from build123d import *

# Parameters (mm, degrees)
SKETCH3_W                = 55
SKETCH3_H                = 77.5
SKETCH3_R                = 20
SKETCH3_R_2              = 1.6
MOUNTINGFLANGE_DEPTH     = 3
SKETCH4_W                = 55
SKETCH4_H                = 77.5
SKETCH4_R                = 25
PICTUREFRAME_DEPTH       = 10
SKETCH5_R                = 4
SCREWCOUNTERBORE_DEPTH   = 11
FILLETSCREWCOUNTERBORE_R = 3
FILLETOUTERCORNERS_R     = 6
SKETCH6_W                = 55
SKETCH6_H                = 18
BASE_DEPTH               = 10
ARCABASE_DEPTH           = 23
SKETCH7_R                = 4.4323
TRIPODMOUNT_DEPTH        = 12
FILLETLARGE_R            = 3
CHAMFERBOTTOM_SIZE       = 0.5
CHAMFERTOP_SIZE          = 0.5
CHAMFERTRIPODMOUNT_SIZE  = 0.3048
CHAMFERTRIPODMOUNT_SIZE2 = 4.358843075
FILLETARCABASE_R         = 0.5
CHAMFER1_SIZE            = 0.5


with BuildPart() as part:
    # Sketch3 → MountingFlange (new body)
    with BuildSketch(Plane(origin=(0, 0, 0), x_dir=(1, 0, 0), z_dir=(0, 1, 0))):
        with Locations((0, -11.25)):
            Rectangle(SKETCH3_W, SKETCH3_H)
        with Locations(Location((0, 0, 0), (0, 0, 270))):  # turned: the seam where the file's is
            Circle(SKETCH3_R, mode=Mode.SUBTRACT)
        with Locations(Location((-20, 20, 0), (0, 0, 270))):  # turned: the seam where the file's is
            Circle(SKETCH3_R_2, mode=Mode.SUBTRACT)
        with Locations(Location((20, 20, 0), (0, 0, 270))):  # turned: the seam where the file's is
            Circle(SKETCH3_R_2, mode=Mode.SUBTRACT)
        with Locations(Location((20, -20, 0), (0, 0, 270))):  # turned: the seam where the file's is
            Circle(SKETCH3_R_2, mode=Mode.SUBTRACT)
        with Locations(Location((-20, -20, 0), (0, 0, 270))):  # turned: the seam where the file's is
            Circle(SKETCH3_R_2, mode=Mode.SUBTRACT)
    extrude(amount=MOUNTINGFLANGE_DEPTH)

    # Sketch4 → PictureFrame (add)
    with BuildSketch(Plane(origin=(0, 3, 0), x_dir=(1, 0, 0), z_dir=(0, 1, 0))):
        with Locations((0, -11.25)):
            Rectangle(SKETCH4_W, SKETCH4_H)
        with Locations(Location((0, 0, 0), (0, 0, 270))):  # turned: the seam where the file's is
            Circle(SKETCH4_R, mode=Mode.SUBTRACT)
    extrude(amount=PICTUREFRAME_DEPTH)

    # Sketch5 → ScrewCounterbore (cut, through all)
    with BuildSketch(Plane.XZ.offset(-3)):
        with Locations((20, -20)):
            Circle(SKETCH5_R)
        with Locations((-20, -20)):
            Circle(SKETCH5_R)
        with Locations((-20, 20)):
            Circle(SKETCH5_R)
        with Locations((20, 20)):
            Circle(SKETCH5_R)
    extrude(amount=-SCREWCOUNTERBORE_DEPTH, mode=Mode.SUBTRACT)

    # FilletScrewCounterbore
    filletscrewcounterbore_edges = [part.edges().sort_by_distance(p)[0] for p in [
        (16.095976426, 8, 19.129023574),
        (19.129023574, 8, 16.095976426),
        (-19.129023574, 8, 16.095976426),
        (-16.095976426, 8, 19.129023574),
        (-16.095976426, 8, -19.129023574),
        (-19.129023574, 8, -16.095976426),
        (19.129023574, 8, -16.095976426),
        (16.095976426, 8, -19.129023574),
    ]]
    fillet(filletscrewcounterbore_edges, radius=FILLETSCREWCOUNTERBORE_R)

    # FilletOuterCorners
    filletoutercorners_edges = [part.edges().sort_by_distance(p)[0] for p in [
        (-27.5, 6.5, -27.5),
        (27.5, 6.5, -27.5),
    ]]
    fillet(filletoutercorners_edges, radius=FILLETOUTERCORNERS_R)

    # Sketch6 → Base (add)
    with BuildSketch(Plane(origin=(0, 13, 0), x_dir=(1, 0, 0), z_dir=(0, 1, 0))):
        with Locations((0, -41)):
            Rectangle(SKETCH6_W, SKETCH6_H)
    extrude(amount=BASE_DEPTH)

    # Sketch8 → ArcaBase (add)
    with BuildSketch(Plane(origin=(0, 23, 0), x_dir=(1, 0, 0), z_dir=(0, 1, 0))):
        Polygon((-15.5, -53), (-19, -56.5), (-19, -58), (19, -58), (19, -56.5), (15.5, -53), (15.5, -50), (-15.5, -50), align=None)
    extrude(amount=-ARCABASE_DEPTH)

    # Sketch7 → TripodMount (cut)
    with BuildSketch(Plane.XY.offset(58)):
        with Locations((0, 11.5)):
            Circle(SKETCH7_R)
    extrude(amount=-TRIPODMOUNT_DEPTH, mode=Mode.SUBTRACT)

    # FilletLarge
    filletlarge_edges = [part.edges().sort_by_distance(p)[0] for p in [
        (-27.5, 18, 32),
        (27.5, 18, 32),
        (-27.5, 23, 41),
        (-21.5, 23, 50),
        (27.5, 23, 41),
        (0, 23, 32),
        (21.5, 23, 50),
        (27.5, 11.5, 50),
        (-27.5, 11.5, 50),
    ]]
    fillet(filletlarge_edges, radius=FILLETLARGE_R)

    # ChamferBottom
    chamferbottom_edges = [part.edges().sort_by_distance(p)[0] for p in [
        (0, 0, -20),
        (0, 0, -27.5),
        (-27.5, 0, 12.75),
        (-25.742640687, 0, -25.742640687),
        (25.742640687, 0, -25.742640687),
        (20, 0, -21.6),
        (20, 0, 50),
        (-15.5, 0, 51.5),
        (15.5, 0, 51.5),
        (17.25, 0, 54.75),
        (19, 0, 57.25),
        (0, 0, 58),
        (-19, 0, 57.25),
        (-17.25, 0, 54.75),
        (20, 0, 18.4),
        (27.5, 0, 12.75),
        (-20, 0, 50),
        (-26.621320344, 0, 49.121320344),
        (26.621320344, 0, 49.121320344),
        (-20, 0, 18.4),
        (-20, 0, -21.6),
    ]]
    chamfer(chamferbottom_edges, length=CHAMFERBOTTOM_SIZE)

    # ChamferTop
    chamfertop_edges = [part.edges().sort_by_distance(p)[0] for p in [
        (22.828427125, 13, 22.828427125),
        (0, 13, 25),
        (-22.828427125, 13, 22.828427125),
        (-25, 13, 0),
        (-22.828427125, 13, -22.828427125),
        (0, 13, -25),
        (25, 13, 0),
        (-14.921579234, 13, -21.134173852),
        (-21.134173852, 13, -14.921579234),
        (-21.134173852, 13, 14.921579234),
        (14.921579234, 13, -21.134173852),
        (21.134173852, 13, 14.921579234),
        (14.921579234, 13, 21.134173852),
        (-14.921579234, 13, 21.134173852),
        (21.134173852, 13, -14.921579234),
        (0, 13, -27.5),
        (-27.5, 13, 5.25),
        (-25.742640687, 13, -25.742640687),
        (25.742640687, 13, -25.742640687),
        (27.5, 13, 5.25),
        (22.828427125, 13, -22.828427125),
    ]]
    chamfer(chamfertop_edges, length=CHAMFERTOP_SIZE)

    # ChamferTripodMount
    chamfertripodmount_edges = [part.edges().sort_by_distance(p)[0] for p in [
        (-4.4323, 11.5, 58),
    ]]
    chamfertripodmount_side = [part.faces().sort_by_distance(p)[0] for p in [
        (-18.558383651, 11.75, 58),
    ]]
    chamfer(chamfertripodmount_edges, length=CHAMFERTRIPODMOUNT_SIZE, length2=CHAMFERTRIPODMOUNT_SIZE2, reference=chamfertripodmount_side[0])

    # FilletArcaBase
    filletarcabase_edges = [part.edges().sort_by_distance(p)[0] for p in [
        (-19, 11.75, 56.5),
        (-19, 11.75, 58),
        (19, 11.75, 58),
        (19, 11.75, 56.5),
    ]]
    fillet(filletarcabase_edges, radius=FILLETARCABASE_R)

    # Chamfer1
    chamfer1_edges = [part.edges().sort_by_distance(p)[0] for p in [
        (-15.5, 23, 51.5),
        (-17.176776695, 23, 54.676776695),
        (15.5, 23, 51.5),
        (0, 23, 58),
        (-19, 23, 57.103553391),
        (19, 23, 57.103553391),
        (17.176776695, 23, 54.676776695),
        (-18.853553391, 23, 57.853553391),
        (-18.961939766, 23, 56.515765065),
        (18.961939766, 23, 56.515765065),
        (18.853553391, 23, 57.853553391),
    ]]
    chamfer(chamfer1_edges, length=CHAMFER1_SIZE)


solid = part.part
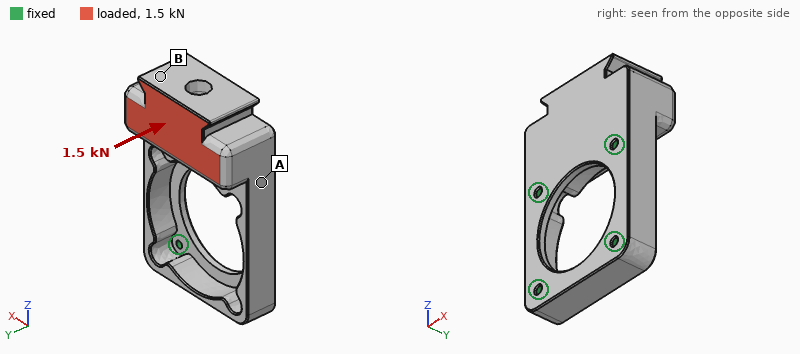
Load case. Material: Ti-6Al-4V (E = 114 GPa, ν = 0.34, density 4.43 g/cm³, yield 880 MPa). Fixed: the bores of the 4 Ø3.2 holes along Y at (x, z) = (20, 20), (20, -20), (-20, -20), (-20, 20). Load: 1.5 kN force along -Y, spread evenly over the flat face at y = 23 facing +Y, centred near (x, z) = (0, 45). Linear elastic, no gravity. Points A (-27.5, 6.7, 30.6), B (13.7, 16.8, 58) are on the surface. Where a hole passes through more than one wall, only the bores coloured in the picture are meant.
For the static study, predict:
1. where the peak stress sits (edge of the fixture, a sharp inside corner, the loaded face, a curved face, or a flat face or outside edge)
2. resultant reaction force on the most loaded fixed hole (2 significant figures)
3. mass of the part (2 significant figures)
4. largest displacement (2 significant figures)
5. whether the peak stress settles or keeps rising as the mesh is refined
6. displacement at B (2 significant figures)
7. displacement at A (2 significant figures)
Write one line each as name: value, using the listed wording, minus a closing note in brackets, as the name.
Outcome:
where the peak stress sits: edge of the fixture
resultant reaction force on the most loaded fixed hole: 1.4 kN
mass of the part: 200 g
largest displacement: 0.12 mm
whether the peak stress settles or keeps rising as the mesh is refined: keeps rising
displacement at B: 0.11 mm
displacement at A: 0.028 mm
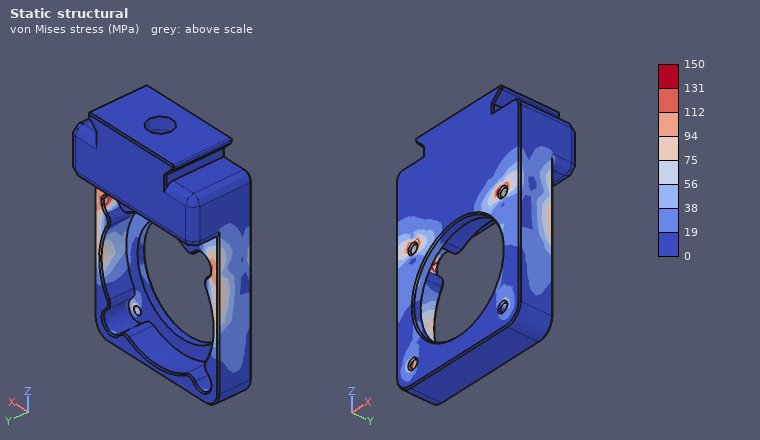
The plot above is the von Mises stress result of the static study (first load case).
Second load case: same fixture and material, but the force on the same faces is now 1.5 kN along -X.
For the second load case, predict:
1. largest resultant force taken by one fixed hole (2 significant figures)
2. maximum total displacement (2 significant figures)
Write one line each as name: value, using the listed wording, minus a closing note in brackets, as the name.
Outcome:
largest resultant force taken by one fixed hole: 1.4 kN
maximum total displacement: 13 µm
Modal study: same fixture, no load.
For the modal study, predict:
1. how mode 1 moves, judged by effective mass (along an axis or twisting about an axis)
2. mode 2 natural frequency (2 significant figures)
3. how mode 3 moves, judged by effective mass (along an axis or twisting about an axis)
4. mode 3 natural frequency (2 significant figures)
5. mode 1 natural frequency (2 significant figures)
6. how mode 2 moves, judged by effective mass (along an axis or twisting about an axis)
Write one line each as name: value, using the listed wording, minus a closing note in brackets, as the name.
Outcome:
how mode 1 moves, judged by effective mass: along Y
mode 2 natural frequency: 6600 Hz
how mode 3 moves, judged by effective mass: along X
mode 3 natural frequency: 8400 Hz
mode 1 natural frequency: 1900 Hz
how mode 2 moves, judged by effective mass: along X
